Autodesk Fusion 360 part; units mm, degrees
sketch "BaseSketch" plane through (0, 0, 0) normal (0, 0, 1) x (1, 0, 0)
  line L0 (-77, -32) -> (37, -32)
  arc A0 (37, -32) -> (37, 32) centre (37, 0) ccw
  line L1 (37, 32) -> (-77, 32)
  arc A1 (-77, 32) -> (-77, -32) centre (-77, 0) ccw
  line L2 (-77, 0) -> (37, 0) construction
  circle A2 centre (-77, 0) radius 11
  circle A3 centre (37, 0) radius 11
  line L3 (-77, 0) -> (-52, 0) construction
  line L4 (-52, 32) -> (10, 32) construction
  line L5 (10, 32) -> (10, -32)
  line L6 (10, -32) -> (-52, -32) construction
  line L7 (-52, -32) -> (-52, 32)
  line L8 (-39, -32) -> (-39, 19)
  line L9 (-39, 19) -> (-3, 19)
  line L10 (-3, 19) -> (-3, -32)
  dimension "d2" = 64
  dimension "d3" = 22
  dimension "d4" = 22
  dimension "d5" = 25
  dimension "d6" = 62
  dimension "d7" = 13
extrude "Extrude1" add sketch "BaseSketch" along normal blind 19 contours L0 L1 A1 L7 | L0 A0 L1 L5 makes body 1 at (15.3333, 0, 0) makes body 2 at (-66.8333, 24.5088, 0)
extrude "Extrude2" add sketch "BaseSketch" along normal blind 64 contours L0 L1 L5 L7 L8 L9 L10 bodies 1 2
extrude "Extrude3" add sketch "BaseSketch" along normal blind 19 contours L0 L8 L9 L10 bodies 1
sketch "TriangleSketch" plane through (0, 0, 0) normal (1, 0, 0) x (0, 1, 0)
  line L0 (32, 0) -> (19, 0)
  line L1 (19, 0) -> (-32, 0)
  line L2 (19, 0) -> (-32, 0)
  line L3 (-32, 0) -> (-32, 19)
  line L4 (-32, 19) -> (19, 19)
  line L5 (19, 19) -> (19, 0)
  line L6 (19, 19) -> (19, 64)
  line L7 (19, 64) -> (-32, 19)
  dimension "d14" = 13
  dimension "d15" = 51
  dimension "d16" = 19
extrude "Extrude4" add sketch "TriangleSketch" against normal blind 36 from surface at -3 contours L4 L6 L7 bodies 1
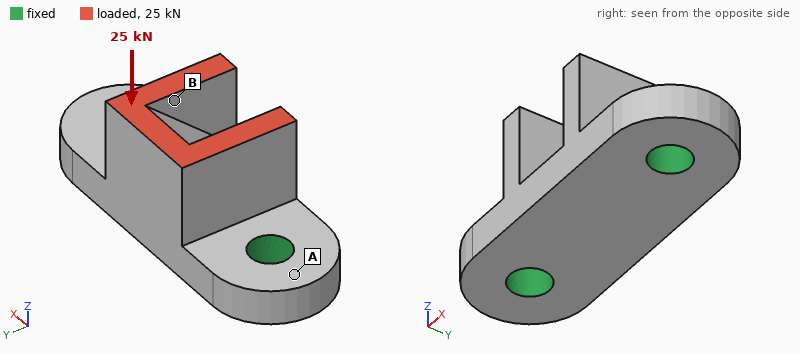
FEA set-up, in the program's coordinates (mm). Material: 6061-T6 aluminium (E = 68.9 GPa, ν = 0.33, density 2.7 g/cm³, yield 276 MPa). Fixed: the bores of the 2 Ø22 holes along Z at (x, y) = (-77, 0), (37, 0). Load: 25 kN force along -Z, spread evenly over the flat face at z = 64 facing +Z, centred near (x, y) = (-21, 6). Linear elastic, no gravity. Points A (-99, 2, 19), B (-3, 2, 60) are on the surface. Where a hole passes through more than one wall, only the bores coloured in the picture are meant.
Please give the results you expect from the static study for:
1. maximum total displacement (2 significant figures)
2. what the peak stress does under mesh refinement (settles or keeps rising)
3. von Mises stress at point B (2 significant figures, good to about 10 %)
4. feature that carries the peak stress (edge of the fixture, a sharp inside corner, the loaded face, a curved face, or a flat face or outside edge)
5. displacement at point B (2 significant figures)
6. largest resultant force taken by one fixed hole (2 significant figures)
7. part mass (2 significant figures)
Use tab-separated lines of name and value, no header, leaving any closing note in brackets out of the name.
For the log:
maximum total displacement	55 µm
what the peak stress does under mesh refinement	keeps rising
von Mises stress at point B	13 MPa
feature that carries the peak stress	edge of the fixture
displacement at point B	39 µm
largest resultant force taken by one fixed hole	13 kN
part mass	870 g
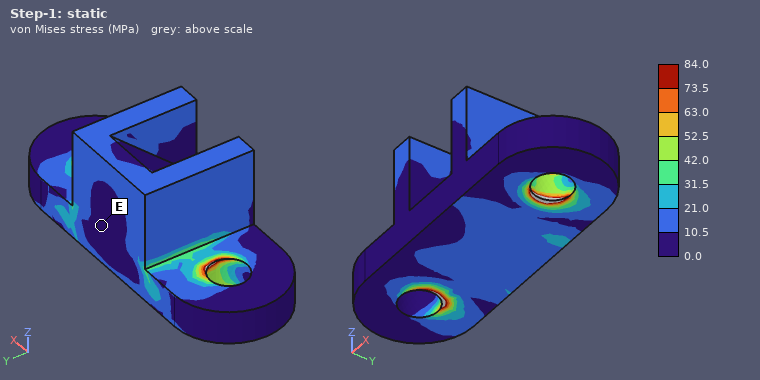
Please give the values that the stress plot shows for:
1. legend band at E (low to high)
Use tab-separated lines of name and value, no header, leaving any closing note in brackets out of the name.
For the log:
legend band at E	0.0 to 10.5 MPa
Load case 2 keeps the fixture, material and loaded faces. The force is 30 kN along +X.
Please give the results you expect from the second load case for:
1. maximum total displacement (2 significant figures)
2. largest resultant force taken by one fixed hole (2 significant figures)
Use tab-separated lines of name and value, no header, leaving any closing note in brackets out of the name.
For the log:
maximum total displacement	0.22 mm
largest resultant force taken by one fixed hole	25 kN
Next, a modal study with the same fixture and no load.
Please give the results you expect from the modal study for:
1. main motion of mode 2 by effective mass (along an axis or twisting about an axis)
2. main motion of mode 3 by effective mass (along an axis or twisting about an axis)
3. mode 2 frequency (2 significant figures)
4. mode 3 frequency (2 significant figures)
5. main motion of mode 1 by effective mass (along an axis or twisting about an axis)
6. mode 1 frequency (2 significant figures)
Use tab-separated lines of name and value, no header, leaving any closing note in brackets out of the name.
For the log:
main motion of mode 2 by effective mass	along Z
main motion of mode 3 by effective mass	along X
mode 2 frequency	6200 Hz
mode 3 frequency	7000 Hz
main motion of mode 1 by effective mass	along Y
mode 1 frequency	3500 Hz
